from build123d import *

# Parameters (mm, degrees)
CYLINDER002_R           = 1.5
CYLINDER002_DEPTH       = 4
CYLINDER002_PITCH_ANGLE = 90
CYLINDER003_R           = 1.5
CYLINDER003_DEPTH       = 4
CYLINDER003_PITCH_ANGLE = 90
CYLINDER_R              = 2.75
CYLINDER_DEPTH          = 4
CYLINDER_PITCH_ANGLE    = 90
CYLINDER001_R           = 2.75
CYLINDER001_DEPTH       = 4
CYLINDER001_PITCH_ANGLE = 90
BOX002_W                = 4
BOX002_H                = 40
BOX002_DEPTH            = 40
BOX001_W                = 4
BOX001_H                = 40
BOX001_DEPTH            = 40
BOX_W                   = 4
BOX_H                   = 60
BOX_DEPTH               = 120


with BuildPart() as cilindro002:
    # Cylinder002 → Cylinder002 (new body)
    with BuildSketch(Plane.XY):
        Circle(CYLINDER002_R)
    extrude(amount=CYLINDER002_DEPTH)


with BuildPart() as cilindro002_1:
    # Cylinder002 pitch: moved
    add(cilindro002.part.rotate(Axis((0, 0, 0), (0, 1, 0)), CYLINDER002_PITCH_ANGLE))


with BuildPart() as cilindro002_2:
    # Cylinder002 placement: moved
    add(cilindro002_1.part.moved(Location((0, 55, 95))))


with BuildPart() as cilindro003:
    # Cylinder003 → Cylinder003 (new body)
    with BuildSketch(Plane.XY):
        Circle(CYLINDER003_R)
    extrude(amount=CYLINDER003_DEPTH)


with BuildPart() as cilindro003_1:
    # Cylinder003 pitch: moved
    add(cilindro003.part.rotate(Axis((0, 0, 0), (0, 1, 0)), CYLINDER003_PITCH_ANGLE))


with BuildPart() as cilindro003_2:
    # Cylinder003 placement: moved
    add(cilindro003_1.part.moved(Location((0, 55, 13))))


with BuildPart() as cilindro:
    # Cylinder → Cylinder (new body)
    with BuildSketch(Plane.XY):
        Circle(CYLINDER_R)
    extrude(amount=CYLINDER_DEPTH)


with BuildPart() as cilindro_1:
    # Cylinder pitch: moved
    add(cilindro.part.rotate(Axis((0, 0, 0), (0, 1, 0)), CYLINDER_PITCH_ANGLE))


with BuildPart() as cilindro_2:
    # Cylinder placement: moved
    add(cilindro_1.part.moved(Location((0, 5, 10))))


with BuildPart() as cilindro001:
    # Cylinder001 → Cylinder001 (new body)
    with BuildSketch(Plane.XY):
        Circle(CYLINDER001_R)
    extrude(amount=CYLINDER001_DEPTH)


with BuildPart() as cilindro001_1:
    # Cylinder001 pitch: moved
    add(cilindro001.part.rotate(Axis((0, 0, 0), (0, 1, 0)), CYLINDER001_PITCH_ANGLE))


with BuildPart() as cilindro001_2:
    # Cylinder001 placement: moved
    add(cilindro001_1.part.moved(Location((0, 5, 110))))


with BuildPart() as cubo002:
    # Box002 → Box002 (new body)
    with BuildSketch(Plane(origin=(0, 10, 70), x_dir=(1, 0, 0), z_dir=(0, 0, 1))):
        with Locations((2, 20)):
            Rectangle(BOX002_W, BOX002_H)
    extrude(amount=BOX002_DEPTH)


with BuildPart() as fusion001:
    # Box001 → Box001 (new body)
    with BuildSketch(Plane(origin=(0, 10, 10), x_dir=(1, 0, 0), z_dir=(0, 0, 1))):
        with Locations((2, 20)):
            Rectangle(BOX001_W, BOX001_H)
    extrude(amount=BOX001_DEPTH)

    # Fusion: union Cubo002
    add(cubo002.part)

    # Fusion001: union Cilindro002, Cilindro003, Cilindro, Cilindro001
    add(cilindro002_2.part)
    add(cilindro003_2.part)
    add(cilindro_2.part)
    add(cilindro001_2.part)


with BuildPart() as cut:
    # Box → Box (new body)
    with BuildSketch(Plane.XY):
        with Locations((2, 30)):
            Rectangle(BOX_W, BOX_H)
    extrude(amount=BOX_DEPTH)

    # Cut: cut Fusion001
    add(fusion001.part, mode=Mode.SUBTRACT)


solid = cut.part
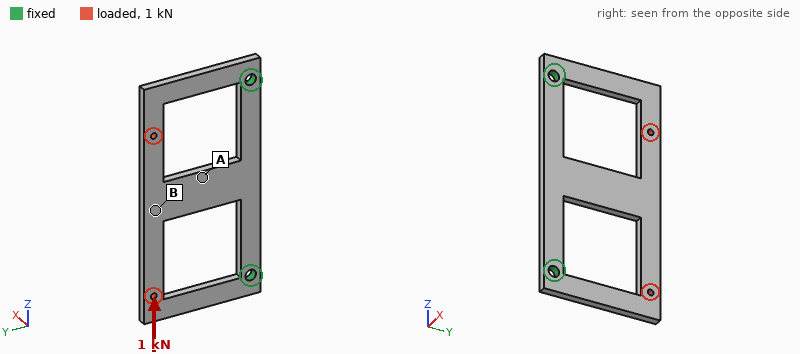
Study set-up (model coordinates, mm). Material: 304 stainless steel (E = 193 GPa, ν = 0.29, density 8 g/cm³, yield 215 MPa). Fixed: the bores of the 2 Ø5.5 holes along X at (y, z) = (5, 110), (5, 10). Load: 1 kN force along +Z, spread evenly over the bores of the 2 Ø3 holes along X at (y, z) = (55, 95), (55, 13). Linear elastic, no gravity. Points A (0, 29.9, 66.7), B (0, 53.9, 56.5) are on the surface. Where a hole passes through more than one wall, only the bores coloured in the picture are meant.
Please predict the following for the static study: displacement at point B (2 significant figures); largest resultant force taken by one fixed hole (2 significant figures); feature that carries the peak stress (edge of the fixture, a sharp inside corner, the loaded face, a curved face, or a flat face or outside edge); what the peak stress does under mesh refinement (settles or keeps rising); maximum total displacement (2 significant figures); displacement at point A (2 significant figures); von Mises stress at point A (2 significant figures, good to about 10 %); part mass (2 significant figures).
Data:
52 µm
660 N
a sharp inside corner
keeps rising
57 µm
28 µm
9.9 MPa
130 g
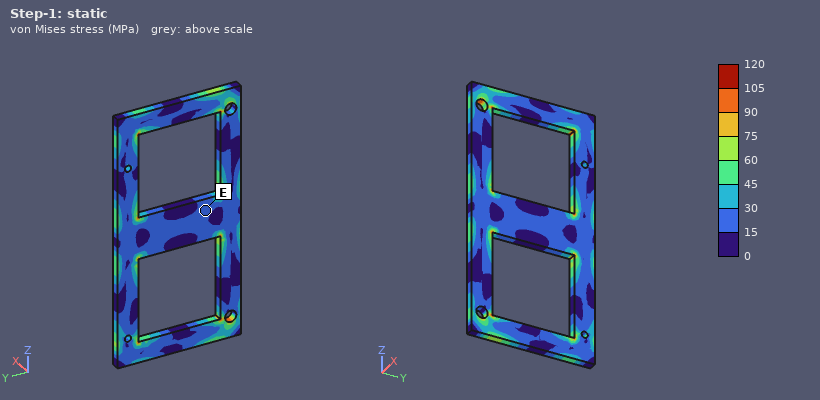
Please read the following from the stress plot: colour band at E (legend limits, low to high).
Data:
15 to 30 MPa
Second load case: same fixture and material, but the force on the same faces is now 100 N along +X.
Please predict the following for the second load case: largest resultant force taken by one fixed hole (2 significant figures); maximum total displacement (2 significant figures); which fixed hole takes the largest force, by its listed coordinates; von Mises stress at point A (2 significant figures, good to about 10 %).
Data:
54 N
0.18 mm
(5, 10)
14 MPa
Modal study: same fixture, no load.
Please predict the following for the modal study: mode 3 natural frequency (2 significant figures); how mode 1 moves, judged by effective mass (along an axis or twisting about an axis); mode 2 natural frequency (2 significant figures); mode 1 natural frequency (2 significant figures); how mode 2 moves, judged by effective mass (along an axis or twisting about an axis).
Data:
1600 Hz
along X
1100 Hz
560 Hz
twisting about Y
